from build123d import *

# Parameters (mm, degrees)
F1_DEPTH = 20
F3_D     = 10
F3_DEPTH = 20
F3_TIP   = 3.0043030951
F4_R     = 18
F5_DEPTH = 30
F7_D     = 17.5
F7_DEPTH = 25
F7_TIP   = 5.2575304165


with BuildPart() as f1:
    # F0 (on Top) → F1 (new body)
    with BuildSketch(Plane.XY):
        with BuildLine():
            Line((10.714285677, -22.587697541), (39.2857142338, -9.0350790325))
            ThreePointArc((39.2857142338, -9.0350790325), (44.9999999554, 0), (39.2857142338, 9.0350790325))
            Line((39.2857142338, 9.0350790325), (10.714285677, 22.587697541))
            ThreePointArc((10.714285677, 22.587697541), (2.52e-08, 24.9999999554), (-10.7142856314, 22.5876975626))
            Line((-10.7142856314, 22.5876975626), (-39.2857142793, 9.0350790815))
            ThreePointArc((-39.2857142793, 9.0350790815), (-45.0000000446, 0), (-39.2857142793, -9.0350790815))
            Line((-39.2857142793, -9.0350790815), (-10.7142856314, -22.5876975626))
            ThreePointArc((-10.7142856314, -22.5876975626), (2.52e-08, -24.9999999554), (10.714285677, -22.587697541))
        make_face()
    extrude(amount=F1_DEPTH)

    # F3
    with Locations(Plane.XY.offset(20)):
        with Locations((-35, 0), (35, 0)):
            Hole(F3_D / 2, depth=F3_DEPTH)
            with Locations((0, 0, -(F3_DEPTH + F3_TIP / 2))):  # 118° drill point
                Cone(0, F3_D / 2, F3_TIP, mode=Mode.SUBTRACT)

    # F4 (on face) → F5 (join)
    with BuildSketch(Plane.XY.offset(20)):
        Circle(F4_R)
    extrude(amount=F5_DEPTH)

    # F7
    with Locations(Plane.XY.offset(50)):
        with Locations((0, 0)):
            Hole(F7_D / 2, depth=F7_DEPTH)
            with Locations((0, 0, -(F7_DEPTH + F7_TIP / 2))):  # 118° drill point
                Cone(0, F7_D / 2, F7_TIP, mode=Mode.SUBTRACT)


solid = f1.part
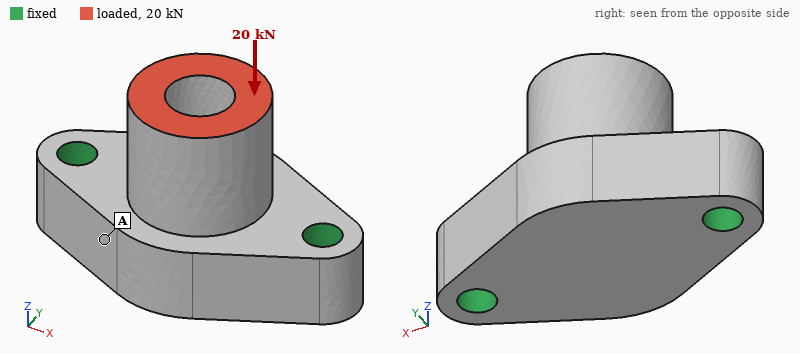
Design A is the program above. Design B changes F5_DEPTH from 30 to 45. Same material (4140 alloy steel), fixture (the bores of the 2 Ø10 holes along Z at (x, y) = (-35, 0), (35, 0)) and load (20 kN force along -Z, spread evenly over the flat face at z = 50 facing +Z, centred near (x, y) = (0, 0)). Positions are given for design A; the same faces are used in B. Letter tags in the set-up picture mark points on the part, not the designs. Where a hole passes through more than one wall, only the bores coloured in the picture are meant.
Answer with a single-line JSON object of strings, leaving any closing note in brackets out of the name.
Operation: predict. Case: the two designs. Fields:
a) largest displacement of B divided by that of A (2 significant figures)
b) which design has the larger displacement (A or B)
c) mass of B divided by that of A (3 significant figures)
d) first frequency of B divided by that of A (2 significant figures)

{"largest displacement of B divided by that of A": "1.2", "which design has the larger displacement": "B", "mass of B divided by that of A": "1.14", "first frequency of B divided by that of A": "0.67"}
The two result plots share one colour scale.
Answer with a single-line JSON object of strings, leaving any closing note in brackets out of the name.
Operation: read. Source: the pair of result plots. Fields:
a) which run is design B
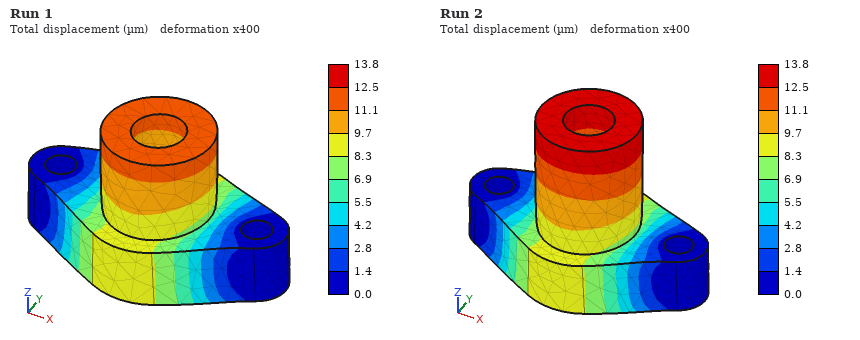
{"which run is design B": "Run 2"}
